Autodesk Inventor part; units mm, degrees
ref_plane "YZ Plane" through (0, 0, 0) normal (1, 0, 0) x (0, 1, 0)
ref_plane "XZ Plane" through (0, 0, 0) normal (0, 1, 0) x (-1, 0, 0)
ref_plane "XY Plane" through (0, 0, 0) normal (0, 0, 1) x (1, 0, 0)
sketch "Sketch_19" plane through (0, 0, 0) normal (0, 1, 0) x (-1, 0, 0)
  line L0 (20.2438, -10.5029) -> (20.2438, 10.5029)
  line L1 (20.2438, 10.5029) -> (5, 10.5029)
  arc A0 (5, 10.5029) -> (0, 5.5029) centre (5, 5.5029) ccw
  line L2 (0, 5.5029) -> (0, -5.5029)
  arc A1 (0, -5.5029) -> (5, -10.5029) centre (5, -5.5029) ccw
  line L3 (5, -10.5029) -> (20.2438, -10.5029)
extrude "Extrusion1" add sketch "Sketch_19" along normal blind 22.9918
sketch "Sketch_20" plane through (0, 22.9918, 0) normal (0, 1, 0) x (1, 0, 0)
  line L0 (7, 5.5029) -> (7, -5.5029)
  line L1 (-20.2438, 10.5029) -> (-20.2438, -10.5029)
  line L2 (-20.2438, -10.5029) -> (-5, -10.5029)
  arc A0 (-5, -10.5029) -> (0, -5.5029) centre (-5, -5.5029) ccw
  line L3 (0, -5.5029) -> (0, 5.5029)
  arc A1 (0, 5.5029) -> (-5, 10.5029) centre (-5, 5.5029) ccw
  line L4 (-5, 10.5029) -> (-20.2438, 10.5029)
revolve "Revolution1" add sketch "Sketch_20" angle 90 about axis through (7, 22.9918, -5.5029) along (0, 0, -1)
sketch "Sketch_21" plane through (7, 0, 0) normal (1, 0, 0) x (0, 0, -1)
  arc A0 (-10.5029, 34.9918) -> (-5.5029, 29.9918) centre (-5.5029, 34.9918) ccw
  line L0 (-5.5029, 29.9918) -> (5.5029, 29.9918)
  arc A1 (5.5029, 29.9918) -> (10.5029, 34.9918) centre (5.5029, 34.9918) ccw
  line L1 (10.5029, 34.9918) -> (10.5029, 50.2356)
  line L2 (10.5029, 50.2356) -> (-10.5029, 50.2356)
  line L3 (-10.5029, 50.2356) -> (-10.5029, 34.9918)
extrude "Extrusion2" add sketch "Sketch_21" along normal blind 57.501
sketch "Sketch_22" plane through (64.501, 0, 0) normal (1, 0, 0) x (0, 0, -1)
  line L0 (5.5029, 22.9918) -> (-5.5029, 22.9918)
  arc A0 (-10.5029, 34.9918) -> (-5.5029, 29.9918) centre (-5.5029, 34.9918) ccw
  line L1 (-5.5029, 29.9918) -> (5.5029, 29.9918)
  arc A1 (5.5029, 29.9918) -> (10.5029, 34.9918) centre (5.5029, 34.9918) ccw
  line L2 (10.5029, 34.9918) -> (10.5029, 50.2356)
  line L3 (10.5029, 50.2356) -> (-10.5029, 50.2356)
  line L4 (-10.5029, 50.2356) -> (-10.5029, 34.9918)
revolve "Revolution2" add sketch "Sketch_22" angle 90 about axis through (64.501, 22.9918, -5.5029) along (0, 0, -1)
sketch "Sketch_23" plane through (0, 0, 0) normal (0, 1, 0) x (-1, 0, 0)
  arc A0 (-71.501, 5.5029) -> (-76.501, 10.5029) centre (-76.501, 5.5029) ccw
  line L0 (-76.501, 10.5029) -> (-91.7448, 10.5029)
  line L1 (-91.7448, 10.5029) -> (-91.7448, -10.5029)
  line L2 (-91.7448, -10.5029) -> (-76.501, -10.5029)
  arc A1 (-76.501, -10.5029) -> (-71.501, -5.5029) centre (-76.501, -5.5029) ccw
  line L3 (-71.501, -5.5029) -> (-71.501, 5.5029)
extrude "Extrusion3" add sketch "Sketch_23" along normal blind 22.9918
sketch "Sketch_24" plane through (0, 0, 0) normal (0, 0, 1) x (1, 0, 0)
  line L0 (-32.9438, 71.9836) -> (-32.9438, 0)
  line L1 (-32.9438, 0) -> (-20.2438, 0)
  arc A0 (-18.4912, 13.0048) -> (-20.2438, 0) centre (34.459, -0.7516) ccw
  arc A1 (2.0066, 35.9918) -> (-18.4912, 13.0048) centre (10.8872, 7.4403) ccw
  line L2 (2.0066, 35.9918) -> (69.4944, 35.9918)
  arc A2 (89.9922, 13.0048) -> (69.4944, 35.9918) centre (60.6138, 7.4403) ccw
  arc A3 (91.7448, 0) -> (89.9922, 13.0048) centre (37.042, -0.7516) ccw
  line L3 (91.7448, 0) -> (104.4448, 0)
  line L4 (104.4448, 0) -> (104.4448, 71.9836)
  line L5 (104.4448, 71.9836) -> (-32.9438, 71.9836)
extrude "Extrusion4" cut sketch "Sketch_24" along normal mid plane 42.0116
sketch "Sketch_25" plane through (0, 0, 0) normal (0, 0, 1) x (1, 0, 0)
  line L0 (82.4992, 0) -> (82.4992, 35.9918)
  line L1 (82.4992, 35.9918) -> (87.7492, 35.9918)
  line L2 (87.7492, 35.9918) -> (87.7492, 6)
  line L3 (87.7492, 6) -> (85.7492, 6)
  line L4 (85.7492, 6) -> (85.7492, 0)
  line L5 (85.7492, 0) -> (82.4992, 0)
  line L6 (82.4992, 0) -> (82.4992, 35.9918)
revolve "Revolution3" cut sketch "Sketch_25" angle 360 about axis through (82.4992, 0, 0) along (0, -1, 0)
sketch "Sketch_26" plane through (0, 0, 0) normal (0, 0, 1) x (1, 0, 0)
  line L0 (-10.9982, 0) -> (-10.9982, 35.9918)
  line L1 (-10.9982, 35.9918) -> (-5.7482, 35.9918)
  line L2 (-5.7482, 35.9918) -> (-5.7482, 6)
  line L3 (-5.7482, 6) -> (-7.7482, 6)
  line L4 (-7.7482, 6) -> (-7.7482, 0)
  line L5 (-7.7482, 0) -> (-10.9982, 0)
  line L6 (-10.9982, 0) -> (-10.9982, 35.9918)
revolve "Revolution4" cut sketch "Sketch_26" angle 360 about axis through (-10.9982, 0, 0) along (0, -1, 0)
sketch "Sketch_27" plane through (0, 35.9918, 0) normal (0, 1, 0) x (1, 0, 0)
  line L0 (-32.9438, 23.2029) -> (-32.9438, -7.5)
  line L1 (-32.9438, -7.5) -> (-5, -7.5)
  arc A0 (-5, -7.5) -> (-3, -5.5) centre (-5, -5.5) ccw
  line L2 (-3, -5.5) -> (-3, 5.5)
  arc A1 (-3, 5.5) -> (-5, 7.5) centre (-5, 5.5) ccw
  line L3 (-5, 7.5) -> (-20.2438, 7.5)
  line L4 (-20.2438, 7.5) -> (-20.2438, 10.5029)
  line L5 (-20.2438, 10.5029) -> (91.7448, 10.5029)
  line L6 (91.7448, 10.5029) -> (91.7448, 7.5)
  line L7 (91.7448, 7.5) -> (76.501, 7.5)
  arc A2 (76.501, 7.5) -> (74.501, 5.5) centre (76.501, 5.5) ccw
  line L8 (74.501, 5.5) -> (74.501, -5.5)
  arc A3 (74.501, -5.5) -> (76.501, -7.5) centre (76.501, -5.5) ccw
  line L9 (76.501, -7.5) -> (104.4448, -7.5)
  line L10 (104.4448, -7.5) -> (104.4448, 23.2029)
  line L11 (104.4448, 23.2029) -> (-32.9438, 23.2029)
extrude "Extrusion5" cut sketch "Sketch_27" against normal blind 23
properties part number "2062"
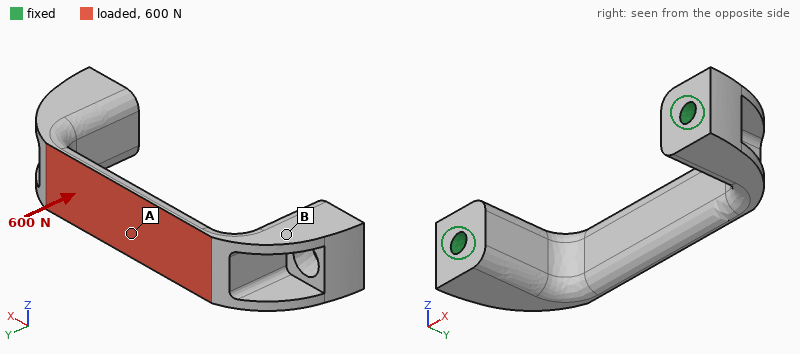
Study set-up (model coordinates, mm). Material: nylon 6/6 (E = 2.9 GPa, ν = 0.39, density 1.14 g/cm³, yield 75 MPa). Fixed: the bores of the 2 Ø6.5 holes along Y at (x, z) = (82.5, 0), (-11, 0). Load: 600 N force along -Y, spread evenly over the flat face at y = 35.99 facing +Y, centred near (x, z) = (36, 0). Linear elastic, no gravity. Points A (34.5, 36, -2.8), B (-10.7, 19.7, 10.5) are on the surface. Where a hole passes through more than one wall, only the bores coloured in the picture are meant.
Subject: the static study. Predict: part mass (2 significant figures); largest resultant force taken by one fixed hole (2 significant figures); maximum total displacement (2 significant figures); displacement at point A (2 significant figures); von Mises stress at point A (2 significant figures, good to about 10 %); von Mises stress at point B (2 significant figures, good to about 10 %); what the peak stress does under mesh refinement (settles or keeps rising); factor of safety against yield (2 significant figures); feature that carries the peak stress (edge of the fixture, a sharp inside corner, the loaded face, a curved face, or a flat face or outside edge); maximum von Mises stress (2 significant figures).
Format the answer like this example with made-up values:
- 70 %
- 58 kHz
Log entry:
- 26 g
- 390 N
- 0.98 mm
- 0.93 mm
- 21 MPa
- 3.8 MPa
- settles
- 2.3
- a curved face
- 32 MPa
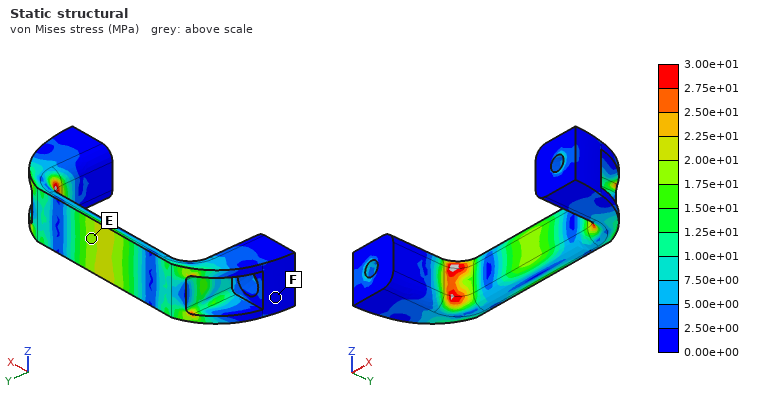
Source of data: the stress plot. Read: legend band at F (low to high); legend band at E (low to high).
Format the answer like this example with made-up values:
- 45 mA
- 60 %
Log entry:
- 0.00e+00 to 2.50e+00 MPa
- 1.75e+01 to 2.00e+01 MPa
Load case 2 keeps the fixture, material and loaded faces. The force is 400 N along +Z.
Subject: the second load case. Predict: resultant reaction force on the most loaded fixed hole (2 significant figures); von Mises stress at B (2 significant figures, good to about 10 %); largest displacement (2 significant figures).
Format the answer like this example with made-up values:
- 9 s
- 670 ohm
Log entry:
- 200 N
- 5.5 MPa
- 0.73 mm
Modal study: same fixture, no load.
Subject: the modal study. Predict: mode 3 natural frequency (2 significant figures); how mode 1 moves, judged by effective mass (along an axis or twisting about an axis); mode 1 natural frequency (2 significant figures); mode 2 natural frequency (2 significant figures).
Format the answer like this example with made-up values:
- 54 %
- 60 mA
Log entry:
- 1500 Hz
- along Z
- 1300 Hz
- 1500 Hz
